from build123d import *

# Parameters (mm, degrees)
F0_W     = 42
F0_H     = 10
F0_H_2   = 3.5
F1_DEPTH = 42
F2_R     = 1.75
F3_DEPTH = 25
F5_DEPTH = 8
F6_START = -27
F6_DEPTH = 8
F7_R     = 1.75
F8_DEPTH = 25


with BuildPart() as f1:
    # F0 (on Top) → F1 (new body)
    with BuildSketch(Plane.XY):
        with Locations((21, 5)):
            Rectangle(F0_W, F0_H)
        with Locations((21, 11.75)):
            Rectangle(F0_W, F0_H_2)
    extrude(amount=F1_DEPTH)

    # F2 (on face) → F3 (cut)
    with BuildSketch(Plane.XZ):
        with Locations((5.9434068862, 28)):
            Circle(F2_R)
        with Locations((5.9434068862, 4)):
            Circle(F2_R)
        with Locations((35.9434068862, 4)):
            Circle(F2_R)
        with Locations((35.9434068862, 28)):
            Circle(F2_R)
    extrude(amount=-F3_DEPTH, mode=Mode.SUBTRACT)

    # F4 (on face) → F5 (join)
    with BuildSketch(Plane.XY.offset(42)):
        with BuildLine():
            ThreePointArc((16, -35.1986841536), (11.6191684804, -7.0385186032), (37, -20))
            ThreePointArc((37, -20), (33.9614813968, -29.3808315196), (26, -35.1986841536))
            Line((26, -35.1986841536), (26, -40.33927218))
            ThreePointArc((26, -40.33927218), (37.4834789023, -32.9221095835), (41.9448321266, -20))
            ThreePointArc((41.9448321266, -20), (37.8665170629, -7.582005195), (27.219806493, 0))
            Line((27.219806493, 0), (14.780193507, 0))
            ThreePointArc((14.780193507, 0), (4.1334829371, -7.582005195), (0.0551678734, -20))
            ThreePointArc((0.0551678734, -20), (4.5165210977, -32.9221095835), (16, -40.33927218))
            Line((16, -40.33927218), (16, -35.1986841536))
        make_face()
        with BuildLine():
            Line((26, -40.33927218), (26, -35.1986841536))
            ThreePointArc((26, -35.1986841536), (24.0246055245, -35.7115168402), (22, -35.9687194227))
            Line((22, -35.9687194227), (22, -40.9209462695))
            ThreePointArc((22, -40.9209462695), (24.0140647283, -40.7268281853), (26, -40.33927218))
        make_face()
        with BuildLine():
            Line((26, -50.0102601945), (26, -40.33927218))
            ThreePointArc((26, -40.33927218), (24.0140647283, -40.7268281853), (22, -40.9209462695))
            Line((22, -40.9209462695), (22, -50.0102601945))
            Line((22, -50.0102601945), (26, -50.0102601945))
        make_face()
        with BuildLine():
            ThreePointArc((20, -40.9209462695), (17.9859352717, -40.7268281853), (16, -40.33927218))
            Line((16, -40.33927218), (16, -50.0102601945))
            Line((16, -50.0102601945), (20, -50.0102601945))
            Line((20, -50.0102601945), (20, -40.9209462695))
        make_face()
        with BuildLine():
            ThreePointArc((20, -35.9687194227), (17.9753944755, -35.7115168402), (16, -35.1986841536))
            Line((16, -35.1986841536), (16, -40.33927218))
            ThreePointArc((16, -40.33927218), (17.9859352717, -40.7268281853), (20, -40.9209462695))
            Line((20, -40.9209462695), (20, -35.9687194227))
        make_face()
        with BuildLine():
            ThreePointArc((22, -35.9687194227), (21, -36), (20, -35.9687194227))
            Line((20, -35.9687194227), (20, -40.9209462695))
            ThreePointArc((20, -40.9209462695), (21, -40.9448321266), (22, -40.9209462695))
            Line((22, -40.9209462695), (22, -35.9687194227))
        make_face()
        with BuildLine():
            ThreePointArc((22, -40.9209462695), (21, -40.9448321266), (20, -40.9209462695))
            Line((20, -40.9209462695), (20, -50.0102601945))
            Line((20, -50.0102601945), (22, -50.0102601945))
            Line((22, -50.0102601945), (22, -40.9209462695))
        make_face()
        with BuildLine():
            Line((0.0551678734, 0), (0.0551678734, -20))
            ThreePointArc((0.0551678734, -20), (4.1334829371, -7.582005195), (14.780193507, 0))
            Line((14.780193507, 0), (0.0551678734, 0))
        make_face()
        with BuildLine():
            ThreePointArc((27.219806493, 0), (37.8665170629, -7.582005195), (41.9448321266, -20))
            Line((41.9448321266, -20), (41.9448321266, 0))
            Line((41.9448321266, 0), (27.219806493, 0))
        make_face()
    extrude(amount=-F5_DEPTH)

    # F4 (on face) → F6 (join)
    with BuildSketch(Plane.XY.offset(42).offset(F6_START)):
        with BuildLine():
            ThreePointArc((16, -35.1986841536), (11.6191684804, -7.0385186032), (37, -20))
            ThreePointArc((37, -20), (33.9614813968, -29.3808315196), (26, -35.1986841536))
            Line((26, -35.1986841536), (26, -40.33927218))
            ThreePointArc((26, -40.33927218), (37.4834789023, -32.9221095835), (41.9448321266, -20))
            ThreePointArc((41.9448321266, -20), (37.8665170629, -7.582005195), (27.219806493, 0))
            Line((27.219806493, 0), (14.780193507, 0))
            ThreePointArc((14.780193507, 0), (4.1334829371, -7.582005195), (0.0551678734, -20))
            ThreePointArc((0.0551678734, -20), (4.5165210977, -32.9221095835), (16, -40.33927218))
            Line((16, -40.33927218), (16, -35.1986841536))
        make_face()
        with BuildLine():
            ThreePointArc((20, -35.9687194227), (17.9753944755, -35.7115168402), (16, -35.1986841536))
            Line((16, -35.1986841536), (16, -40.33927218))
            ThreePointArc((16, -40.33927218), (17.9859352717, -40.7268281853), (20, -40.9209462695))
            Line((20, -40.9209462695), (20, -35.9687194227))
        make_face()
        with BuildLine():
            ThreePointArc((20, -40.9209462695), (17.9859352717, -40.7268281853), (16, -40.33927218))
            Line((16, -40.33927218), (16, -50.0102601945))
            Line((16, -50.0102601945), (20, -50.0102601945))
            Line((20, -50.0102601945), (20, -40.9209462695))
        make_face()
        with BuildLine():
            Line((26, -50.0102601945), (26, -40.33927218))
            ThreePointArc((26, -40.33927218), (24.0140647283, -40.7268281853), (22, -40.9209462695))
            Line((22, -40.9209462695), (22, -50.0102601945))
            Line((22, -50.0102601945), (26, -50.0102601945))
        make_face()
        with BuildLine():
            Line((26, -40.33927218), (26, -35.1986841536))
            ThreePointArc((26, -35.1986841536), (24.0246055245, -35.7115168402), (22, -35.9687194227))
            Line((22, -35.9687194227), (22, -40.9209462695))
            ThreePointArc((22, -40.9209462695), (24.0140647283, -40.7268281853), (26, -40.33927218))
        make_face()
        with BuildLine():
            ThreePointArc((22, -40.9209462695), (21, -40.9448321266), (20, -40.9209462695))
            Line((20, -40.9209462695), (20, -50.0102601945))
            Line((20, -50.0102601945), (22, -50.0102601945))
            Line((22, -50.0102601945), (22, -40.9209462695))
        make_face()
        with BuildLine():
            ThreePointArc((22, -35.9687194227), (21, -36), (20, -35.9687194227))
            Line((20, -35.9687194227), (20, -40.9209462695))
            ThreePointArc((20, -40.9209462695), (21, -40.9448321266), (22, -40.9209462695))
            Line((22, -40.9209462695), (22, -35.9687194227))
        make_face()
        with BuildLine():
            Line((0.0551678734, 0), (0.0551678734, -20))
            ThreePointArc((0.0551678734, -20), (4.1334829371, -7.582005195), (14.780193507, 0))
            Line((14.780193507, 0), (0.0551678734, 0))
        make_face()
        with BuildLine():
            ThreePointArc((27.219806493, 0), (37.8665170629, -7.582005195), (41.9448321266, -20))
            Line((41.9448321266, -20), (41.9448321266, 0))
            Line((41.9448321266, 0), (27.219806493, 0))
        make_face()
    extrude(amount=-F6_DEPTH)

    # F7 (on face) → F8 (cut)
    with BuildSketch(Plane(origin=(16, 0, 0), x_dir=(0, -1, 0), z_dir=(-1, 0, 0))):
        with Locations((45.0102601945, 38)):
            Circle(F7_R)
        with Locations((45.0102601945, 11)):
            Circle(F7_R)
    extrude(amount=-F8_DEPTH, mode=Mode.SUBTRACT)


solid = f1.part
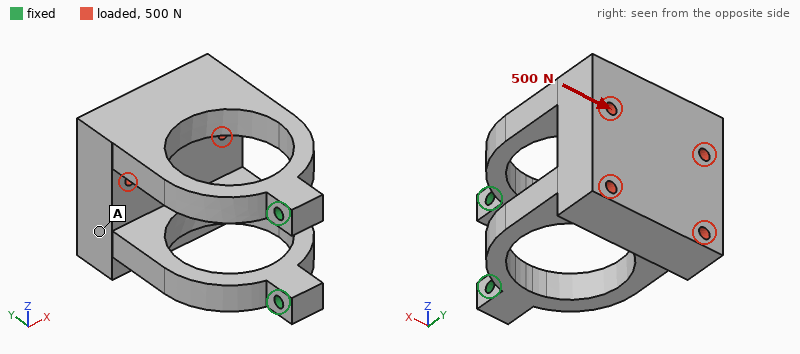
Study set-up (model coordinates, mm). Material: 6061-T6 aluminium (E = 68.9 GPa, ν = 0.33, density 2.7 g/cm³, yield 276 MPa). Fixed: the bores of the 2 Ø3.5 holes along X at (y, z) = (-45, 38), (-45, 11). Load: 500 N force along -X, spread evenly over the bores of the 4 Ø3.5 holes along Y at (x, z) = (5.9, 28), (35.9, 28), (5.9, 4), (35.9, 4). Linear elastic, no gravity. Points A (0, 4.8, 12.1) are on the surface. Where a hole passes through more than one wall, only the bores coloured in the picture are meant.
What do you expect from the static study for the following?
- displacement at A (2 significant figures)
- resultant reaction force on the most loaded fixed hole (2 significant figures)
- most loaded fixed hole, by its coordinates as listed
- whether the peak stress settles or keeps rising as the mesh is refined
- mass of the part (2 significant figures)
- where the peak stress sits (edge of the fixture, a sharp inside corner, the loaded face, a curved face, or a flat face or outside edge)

0.37 mm
330 N
(-45, 11)
keeps rising
98 g
edge of the fixture
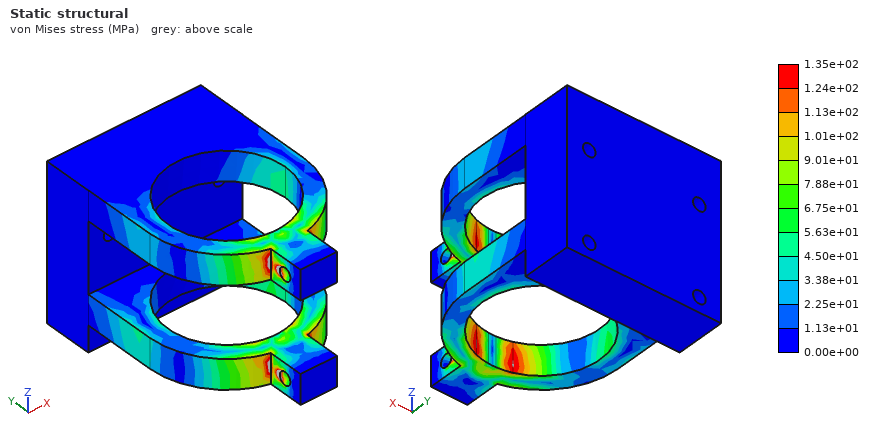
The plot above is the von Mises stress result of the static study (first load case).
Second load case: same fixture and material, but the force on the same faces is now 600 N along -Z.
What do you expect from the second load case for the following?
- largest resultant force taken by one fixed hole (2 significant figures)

760 N
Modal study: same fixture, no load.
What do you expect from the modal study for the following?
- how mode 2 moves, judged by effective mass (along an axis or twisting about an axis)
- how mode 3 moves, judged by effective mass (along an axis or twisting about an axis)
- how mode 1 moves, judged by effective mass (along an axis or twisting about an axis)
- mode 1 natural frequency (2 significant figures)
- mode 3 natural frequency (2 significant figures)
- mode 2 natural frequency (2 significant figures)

along Z
twisting about Y
along X
680 Hz
2200 Hz
1100 Hz
